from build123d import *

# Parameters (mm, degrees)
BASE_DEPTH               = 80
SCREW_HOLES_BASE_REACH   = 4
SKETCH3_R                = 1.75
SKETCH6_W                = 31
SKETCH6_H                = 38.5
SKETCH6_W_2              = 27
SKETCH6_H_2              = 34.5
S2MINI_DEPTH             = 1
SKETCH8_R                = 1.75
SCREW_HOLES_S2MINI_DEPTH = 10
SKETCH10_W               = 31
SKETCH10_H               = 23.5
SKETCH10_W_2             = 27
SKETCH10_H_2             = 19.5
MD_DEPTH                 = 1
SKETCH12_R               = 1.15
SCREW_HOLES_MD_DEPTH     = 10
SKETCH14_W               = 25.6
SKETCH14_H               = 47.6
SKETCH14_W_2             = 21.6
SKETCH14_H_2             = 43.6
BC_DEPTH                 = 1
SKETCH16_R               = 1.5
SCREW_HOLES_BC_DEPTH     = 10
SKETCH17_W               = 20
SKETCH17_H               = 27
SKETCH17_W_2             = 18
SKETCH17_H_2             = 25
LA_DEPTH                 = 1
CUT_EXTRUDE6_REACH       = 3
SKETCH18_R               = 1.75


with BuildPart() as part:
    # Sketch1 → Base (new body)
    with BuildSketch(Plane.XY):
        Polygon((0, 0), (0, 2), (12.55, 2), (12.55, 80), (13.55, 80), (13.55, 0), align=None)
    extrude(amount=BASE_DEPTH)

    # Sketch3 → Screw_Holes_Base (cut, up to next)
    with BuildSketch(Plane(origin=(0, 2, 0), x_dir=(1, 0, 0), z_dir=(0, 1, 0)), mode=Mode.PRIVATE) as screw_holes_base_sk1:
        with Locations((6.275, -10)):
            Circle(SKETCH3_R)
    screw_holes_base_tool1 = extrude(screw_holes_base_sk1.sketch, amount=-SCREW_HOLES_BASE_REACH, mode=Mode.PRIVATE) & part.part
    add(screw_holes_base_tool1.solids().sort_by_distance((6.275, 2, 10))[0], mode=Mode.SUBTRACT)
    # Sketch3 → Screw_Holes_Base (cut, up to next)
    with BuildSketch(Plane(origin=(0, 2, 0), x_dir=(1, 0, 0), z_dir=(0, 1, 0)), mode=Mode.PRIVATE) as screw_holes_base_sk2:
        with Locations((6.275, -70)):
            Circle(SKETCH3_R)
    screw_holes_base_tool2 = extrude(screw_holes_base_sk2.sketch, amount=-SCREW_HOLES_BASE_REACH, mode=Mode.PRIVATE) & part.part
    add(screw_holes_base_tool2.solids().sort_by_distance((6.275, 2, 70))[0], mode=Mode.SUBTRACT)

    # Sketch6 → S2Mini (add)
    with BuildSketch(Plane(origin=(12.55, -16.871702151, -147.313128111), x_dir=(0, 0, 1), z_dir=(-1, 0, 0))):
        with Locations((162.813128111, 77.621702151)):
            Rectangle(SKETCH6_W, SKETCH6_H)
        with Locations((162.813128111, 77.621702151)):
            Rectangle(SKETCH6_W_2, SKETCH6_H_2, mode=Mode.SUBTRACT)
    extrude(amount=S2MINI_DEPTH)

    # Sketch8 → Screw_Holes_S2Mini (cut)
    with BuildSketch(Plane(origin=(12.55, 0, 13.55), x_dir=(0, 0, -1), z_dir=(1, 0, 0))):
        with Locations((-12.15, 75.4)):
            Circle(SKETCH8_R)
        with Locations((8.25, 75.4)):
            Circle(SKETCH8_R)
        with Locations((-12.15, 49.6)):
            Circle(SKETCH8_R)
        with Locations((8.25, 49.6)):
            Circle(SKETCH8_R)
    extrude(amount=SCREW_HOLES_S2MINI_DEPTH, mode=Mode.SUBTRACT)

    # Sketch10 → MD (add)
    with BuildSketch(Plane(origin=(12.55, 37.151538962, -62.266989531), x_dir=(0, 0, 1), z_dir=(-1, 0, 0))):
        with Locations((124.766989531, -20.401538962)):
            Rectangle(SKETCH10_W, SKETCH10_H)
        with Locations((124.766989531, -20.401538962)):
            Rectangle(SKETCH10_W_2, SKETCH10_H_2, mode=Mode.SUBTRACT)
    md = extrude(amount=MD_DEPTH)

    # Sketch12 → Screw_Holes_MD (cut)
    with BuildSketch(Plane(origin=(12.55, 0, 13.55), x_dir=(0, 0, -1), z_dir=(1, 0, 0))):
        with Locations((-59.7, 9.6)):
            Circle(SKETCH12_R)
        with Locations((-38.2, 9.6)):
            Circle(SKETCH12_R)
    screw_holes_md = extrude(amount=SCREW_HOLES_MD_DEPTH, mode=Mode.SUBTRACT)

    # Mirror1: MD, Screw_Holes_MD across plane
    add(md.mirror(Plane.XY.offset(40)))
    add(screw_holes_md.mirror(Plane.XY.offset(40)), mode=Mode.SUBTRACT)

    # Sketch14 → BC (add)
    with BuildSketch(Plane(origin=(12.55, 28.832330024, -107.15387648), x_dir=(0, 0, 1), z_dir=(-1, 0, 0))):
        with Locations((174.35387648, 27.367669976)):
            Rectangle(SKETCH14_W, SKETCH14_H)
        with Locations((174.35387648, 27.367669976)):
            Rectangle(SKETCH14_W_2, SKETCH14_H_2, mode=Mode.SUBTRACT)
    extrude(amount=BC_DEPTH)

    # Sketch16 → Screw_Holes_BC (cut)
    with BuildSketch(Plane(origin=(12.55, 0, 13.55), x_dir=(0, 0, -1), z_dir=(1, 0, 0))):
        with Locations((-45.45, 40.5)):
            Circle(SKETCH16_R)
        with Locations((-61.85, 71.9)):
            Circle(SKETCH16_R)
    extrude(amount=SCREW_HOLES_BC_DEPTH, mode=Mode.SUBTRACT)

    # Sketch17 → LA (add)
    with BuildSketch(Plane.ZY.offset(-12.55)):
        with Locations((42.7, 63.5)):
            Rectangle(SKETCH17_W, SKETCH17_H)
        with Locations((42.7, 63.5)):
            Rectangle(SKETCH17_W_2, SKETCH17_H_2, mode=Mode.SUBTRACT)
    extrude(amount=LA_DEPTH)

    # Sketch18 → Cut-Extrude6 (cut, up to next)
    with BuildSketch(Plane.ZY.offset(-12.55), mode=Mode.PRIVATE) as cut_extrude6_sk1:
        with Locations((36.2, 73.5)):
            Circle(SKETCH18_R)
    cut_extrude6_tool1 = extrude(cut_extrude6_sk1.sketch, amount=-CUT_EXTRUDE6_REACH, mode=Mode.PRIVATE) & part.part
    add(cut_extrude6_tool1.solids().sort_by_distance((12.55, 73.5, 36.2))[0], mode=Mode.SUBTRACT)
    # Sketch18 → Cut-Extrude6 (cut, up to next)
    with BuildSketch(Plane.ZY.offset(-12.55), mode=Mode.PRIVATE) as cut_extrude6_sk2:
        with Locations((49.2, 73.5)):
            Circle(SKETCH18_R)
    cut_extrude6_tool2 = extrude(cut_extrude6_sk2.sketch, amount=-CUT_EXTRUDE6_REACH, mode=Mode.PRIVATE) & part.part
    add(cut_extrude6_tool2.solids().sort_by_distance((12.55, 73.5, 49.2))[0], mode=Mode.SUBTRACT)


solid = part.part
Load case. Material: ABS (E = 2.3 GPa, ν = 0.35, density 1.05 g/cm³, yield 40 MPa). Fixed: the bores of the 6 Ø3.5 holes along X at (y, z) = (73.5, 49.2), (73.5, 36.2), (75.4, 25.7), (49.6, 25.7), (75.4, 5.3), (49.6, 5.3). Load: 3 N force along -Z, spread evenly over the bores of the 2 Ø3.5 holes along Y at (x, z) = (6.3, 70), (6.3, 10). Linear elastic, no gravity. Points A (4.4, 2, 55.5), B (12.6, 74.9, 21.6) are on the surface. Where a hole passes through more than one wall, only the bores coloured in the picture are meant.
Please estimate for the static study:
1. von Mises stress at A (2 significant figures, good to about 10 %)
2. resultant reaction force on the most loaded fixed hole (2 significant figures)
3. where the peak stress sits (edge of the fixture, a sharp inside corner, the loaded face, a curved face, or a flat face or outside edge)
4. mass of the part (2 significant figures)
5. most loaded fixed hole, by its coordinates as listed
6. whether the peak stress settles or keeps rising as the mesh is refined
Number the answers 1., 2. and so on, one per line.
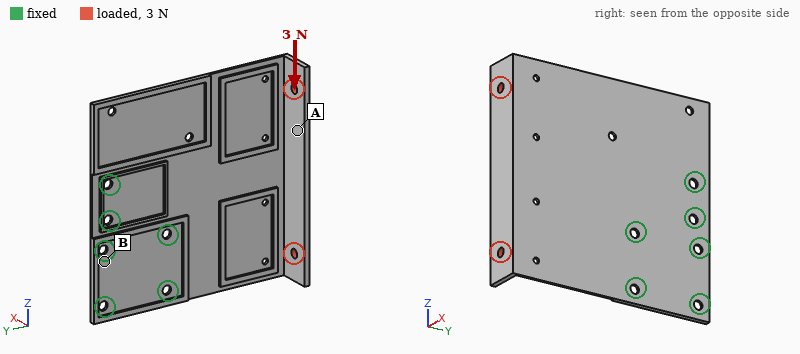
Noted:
1. 0.35 MPa
2. 3.4 N
3. edge of the fixture
4. 9.8 g
5. (49.6, 5.3)
6. keeps rising
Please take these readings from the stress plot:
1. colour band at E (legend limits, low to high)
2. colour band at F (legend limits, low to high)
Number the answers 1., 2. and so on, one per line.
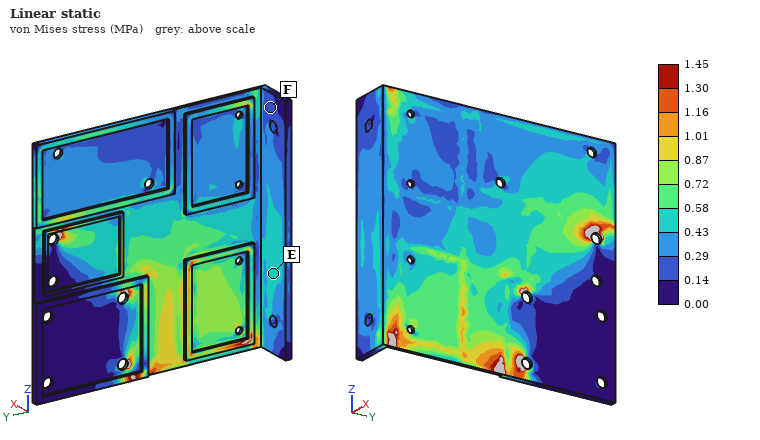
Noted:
1. 0.43 to 0.58 MPa
2. 0.14 to 0.29 MPa
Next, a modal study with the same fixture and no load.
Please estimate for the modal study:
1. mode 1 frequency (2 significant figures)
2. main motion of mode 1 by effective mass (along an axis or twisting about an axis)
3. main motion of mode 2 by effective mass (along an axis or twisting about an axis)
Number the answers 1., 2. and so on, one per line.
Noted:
1. 55 Hz
2. along X
3. twisting about Y
